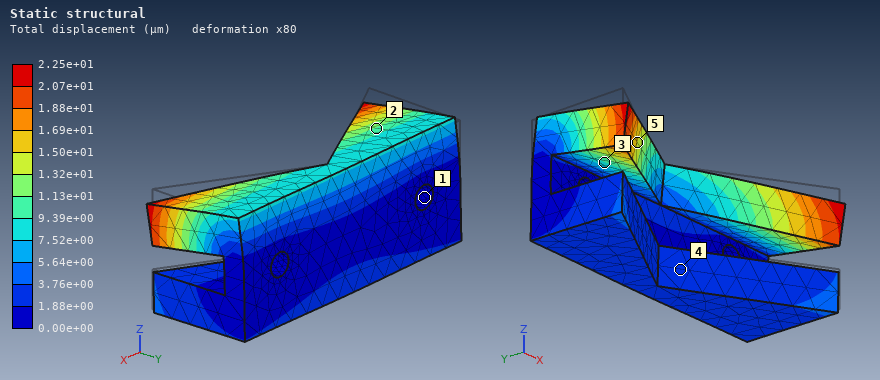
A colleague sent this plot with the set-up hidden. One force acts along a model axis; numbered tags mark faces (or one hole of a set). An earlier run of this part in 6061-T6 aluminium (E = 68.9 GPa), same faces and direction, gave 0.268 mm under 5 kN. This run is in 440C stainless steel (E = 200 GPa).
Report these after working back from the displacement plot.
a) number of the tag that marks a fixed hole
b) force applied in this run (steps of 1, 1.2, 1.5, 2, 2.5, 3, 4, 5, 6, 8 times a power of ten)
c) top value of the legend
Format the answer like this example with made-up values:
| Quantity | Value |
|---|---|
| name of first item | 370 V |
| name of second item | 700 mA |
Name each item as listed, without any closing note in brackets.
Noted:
| Quantity | Value |
|---|---|
| number of the tag that marks a fixed hole | 1 |
| force applied in this run | 1.2 kN |
| top value of the legend | 2.25e+01 µm |
